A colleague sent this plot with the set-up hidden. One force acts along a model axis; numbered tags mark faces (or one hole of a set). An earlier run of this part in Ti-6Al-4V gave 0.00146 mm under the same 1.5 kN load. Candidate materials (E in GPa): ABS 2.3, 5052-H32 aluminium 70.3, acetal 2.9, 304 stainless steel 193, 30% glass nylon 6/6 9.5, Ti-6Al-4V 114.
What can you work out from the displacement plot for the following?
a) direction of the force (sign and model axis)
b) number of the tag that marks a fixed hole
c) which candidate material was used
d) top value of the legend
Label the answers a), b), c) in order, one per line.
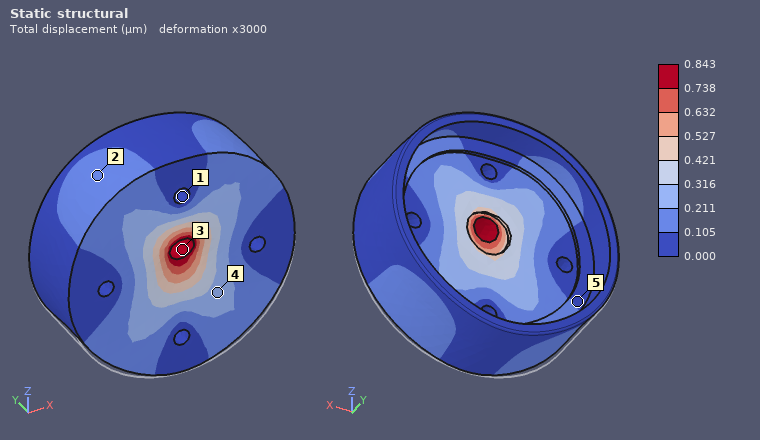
a) +Z
b) 1
c) 304 stainless steel
d) 0.843 µm
